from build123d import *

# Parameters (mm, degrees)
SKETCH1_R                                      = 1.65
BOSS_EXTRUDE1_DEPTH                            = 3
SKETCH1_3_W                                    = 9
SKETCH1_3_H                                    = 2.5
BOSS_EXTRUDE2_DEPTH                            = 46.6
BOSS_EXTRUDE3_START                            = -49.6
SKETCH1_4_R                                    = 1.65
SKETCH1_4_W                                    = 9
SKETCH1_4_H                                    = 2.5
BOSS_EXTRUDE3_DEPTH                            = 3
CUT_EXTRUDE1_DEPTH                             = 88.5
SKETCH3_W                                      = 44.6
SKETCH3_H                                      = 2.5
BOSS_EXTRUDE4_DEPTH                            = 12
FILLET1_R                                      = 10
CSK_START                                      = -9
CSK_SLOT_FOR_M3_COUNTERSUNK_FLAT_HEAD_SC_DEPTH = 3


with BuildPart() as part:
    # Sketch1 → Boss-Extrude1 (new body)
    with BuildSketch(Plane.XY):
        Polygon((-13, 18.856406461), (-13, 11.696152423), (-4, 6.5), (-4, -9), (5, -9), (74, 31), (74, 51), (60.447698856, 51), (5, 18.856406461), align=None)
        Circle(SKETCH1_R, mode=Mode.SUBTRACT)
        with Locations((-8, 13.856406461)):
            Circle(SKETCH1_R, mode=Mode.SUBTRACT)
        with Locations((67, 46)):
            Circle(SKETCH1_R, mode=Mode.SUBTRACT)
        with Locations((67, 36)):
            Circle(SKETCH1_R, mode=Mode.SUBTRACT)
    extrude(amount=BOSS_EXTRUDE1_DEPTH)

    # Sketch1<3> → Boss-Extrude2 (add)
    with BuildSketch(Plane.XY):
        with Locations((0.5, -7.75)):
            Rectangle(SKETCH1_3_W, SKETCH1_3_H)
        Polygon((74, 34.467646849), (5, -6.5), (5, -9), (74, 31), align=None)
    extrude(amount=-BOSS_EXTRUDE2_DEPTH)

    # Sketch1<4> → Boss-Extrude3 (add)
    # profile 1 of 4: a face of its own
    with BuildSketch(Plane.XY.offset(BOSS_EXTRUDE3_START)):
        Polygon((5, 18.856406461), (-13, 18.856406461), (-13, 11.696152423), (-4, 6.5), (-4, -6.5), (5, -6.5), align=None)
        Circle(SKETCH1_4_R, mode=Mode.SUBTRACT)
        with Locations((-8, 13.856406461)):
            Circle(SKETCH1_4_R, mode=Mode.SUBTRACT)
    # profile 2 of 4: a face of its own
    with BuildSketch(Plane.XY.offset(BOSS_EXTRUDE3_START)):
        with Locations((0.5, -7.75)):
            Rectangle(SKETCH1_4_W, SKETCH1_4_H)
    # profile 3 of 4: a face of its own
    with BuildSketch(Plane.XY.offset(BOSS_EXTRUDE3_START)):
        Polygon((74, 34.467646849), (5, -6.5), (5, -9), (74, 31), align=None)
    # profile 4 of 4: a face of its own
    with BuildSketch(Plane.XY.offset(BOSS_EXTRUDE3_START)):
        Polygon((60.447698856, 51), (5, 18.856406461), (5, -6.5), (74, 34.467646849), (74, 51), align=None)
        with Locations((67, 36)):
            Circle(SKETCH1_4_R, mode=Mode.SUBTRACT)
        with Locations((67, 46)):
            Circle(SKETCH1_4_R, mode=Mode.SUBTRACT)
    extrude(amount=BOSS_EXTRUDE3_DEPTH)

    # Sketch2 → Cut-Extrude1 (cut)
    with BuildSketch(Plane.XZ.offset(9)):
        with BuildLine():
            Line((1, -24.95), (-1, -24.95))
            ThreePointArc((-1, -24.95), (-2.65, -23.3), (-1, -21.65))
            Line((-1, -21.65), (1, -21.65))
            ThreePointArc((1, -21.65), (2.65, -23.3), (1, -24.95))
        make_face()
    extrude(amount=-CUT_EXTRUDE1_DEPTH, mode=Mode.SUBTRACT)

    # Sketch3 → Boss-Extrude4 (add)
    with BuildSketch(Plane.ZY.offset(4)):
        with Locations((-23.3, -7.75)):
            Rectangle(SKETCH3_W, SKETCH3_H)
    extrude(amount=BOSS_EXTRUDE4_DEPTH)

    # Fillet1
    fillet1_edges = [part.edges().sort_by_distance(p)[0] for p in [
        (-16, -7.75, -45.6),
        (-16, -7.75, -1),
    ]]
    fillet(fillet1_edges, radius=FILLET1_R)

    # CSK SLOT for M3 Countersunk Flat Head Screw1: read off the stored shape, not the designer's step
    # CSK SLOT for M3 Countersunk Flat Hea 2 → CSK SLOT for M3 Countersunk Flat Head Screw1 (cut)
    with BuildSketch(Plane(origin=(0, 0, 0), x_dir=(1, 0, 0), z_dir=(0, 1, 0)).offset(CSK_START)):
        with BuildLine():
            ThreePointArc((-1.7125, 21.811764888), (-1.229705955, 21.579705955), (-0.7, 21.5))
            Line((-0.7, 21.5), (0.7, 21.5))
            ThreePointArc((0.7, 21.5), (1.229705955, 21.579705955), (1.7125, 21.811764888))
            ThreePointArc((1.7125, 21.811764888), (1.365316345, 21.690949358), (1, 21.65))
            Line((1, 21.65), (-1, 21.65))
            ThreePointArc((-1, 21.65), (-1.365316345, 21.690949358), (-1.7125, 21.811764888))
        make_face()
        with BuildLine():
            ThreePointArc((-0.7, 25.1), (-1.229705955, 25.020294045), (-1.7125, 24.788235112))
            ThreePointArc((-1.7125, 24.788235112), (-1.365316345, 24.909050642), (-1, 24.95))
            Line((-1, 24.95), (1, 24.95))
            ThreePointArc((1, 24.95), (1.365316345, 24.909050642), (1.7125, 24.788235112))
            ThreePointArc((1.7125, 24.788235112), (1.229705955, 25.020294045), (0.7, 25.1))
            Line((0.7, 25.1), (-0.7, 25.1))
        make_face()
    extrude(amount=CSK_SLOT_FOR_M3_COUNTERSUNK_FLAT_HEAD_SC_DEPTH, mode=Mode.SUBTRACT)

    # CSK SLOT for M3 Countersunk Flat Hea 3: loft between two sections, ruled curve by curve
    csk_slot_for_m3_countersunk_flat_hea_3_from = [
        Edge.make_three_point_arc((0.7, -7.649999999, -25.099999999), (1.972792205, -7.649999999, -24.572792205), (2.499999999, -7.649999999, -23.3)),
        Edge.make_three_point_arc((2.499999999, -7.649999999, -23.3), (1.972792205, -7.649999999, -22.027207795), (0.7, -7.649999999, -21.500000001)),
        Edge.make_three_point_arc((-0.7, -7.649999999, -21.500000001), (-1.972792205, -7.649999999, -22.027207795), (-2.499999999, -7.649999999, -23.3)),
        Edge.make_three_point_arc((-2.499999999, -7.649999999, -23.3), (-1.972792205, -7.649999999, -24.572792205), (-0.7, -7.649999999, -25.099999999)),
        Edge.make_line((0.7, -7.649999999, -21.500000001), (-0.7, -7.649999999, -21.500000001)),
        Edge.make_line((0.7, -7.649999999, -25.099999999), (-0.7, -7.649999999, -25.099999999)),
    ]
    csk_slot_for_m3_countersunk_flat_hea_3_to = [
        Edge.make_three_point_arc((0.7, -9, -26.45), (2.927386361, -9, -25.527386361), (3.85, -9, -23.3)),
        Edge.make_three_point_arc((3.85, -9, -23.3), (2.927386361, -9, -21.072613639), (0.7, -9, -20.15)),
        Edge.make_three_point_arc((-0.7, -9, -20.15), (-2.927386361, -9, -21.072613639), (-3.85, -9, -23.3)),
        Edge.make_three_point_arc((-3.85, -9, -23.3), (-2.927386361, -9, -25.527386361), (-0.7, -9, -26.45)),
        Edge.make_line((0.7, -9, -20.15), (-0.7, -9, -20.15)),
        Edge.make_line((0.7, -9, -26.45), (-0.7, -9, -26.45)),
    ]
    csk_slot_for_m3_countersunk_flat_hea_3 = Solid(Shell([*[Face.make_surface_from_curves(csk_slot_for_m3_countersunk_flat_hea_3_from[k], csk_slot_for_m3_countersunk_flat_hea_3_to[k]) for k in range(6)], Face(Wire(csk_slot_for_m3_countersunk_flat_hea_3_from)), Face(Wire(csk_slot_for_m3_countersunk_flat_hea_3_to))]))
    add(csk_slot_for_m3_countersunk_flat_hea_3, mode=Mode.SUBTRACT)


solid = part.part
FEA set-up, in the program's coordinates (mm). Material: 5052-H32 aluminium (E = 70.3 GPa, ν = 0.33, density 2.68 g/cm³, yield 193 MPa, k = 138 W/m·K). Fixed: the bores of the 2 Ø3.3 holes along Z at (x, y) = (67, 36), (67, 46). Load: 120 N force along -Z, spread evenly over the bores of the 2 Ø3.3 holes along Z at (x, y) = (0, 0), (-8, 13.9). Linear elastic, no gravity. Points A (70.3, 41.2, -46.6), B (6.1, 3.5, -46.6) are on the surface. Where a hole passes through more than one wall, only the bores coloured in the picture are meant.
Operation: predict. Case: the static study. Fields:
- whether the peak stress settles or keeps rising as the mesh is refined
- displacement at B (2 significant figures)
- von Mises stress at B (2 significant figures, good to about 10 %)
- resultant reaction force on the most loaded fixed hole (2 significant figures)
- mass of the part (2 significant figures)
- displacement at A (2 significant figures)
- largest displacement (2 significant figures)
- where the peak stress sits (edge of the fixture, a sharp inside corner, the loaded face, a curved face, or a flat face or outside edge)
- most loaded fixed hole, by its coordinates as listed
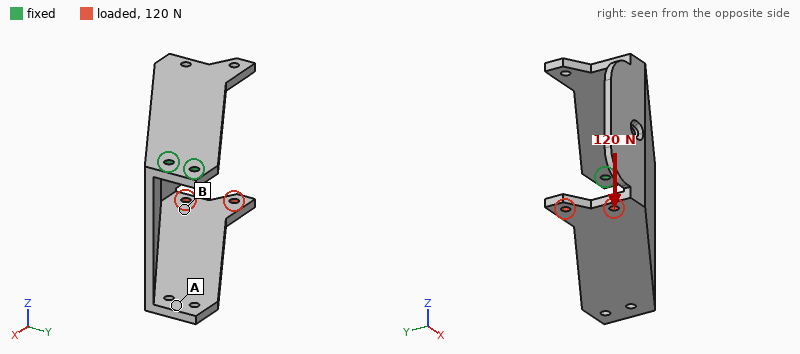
keeps rising
0.96 mm
25 MPa
240 N
67 g
0.48 mm
1.3 mm
edge of the fixture
(67, 36)
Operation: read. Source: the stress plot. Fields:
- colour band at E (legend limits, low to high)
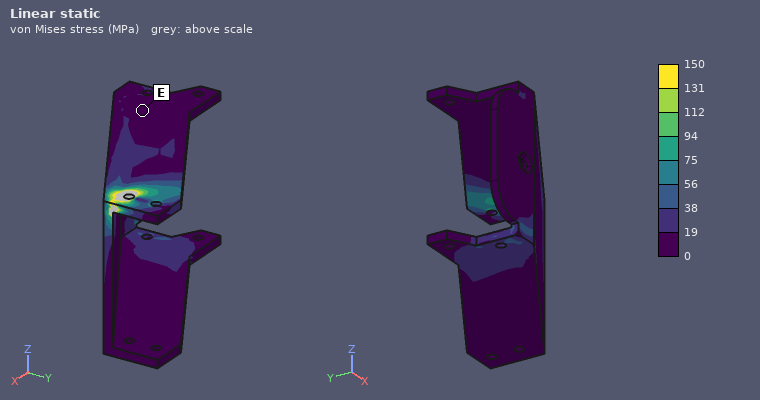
0 to 19 MPa
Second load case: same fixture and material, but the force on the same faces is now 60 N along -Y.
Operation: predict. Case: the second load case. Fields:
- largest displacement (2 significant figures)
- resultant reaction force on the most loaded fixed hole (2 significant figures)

1.2 mm
360 N
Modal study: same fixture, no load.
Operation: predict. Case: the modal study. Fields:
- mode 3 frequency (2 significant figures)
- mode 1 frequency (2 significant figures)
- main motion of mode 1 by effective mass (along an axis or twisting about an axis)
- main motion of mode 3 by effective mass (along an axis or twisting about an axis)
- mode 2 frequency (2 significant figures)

750 Hz
270 Hz
along Y
twisting about Z
320 Hz
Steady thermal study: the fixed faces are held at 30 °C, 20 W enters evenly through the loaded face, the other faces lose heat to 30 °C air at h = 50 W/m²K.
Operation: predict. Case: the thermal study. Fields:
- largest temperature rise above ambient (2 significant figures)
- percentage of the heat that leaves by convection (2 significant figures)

71 K
78 %
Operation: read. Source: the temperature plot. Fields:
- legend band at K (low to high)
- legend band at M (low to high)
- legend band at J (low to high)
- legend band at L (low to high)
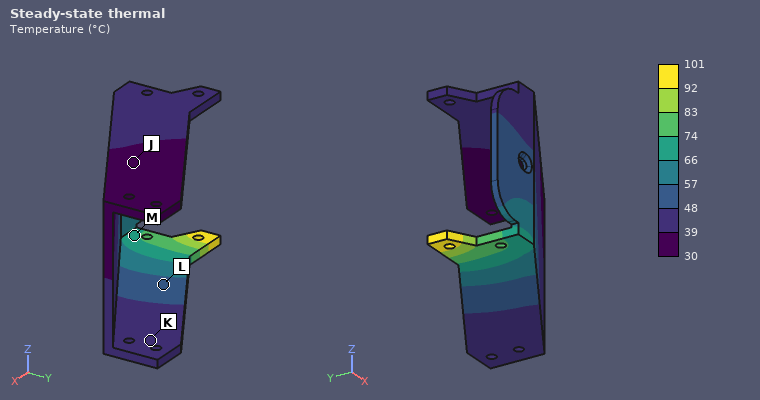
39 to 48 °C
66 to 74 °C
30 to 39 °C
48 to 57 °C
